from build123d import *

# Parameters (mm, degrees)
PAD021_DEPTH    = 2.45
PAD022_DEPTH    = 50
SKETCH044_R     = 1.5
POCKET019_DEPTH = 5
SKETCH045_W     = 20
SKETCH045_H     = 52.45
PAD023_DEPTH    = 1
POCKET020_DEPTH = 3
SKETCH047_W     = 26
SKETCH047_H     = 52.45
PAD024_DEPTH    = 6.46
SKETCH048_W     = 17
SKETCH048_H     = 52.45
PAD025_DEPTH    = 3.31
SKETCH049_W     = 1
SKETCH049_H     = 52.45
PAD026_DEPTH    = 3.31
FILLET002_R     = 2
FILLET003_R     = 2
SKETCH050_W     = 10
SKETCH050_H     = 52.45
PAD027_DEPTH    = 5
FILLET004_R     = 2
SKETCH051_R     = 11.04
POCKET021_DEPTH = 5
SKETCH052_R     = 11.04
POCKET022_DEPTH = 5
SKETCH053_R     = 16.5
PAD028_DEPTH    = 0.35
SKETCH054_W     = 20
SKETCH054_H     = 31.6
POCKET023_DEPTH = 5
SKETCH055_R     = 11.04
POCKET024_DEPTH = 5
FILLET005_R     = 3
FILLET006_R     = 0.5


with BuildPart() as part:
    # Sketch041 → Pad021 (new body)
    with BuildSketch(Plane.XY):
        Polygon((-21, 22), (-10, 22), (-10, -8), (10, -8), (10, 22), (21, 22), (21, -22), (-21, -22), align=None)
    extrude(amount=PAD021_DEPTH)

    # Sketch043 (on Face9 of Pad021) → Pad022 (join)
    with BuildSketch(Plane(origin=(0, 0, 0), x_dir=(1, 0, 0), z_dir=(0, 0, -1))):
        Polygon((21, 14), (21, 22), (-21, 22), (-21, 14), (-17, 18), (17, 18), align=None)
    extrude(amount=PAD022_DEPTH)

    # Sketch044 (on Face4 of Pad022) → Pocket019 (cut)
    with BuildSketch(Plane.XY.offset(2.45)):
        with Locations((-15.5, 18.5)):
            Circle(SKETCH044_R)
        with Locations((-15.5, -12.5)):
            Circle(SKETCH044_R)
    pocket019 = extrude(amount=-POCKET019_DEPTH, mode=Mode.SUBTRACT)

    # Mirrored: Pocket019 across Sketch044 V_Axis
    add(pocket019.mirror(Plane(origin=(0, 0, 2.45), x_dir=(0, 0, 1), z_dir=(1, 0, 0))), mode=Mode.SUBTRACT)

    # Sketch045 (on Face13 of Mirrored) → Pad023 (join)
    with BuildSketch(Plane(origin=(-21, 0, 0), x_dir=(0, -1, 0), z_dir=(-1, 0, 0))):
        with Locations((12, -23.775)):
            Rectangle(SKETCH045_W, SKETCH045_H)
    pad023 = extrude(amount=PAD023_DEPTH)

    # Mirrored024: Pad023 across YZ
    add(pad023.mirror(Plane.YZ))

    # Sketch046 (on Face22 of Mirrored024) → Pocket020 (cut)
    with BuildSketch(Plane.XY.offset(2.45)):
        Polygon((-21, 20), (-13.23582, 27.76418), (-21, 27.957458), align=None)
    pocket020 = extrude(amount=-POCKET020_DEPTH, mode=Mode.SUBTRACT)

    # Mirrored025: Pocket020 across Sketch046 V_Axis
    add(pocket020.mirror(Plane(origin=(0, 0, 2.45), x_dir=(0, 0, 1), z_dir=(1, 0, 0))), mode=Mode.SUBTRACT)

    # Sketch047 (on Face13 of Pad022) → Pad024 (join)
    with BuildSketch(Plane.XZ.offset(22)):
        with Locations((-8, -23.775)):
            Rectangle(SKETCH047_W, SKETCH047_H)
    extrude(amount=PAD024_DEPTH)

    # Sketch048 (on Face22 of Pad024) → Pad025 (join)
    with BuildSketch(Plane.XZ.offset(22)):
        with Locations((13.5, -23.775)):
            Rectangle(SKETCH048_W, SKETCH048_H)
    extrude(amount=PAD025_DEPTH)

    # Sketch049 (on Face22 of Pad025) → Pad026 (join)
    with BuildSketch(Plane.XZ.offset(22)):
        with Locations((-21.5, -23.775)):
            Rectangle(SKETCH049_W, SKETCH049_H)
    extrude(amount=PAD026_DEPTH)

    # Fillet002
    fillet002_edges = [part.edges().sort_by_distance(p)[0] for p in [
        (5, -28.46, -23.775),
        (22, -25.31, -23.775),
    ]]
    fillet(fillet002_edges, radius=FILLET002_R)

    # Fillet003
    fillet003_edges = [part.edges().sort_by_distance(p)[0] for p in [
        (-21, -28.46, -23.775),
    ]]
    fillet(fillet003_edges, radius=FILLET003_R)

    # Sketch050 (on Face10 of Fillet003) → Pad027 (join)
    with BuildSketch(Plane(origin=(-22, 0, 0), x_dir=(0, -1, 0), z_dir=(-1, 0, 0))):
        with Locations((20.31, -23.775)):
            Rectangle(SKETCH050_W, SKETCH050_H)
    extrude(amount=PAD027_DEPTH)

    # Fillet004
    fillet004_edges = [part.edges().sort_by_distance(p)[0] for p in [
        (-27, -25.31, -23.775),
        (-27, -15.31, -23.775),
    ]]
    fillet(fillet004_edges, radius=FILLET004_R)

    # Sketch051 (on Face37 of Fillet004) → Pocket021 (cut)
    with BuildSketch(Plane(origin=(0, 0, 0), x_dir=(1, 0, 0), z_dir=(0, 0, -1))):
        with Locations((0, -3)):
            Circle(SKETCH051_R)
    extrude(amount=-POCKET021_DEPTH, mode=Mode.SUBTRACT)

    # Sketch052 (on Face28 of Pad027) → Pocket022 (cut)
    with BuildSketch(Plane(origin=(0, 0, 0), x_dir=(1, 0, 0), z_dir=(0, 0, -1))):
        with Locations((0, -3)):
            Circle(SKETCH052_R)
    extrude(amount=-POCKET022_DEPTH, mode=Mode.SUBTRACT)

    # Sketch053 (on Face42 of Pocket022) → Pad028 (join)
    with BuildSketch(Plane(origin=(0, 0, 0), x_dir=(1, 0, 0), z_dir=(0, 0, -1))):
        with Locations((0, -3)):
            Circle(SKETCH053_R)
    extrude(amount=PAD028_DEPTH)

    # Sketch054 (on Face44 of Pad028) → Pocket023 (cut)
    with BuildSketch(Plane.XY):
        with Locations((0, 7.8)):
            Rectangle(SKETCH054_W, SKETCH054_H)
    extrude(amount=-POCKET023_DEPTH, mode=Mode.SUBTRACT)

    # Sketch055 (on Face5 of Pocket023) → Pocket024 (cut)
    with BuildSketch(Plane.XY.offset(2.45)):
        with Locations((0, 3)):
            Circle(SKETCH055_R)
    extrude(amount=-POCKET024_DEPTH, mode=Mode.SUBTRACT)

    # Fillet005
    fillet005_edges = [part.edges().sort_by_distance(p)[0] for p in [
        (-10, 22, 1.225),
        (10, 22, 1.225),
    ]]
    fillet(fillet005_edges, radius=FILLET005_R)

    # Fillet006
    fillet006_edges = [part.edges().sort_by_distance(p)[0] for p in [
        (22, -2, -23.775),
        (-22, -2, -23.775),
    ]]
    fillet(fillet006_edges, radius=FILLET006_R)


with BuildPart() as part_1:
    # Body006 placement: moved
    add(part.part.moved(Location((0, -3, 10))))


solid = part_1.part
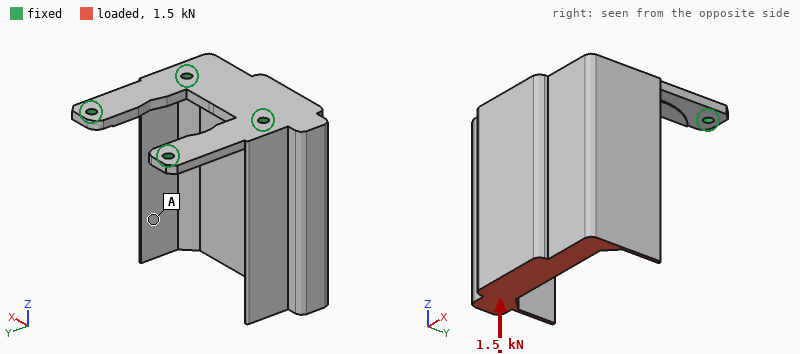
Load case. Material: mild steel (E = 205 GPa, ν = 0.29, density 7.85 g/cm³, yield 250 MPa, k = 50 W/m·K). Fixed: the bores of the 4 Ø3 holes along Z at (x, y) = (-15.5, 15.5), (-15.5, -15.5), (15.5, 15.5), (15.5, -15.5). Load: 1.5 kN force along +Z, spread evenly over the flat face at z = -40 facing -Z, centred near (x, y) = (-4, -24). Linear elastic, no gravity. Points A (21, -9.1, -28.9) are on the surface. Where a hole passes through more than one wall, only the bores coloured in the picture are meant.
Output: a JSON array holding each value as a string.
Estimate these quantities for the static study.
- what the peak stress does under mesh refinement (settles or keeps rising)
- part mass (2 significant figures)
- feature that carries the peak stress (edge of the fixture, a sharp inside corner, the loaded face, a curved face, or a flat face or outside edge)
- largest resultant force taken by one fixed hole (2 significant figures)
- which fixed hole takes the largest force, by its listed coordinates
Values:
["keeps rising", "230 g", "edge of the fixture", "980 N", "(-15.5, -15.5)"]
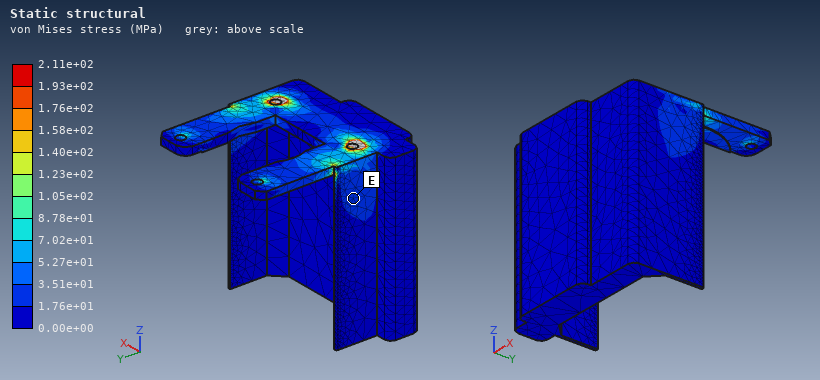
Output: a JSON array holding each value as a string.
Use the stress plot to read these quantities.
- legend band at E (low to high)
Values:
["1.76e+01 to 3.51e+01 MPa"]
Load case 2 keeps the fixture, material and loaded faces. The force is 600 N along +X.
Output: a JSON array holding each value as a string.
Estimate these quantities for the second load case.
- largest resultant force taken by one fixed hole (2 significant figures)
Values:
["960 N"]
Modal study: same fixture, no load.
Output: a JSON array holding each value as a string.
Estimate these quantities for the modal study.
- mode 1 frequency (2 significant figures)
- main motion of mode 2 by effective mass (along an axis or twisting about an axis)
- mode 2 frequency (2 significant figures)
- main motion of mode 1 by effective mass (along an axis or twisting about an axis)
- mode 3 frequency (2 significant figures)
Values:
["770 Hz", "along X", "2700 Hz", "along Y", "5200 Hz"]
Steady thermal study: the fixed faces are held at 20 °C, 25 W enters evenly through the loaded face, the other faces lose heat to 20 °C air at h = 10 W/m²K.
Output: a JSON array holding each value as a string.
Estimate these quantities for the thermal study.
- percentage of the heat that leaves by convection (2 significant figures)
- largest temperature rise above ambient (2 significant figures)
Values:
["20 %", "78 K"]
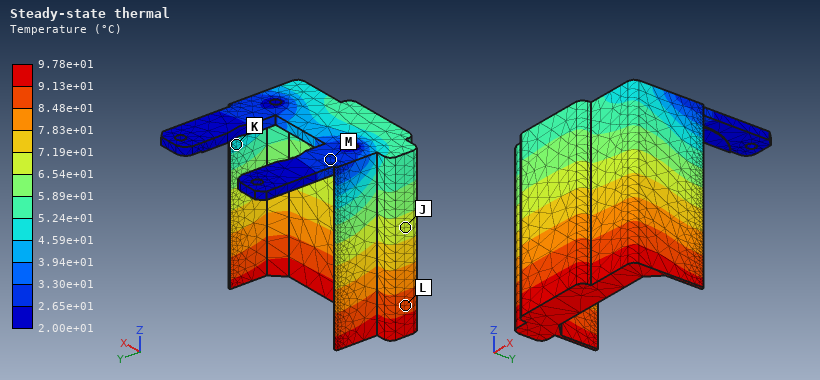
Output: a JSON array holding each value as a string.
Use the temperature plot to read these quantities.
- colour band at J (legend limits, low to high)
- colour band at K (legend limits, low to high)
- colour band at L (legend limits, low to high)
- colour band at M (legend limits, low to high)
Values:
["6.54e+01 to 7.19e+01 °C", "4.59e+01 to 5.24e+01 °C", "8.48e+01 to 9.13e+01 °C", "2.65e+01 to 3.30e+01 °C"]
